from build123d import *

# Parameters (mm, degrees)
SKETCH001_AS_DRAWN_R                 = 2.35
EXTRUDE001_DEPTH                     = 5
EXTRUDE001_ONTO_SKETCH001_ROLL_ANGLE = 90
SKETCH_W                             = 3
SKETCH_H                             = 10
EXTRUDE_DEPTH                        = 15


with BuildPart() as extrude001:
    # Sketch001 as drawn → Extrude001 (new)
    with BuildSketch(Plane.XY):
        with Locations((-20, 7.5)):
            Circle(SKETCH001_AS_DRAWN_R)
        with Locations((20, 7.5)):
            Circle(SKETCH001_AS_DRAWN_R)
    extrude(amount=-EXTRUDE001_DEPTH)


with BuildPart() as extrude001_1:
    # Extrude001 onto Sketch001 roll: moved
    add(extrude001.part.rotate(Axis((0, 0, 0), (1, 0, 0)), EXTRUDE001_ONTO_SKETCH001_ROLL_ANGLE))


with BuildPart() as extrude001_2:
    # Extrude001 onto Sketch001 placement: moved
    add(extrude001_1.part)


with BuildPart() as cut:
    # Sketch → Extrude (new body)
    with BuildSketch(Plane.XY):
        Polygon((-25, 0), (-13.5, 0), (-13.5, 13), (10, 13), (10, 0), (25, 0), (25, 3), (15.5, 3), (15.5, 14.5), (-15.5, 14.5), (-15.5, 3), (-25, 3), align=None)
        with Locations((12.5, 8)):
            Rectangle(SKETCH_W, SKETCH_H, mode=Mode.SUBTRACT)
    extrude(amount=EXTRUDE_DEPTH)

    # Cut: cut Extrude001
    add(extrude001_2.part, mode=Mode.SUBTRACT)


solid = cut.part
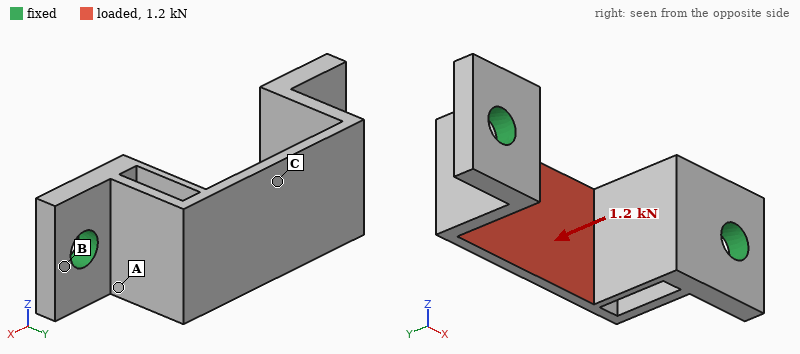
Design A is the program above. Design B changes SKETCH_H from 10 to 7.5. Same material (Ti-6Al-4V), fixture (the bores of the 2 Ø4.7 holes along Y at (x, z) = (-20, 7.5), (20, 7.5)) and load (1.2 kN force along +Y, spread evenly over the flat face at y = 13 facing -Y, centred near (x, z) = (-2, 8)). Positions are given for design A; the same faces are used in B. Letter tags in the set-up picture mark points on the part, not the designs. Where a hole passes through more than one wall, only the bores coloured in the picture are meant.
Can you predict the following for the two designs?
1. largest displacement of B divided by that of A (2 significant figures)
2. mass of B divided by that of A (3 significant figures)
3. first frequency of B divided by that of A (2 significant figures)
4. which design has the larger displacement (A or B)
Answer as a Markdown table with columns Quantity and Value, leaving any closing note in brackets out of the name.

| Quantity | Value |
|---|---|
| largest displacement of B divided by that of A | 0.87 |
| mass of B divided by that of A | 1.05 |
| first frequency of B divided by that of A | 1.1 |
| which design has the larger displacement | A |
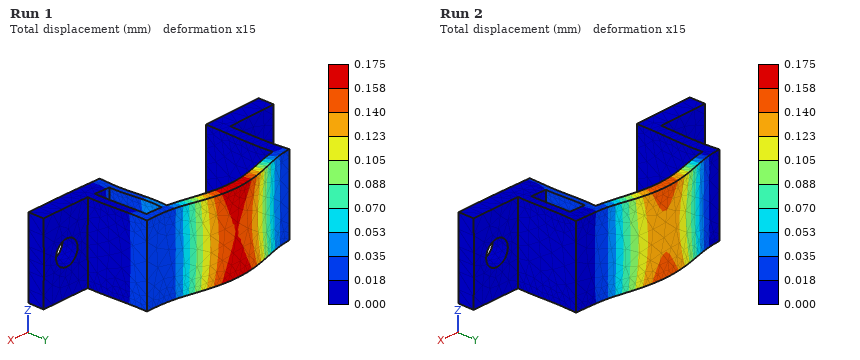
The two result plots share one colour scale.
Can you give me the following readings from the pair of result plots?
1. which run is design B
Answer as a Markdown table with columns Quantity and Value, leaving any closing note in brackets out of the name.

| Quantity | Value |
|---|---|
| which run is design B | Run 2 |
